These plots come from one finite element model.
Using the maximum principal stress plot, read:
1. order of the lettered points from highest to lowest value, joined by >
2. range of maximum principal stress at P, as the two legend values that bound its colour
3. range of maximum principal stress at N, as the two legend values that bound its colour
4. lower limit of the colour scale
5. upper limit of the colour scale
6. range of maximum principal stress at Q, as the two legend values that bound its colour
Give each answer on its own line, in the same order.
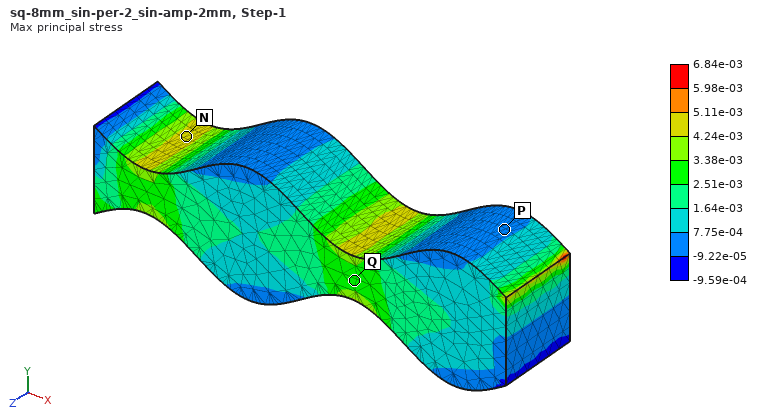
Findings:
N > Q > P
-9.22e-05 to 7.75e-04
4.24e-03 to 5.11e-03
-9.59e-04
6.84e-03
2.51e-03 to 3.38e-03
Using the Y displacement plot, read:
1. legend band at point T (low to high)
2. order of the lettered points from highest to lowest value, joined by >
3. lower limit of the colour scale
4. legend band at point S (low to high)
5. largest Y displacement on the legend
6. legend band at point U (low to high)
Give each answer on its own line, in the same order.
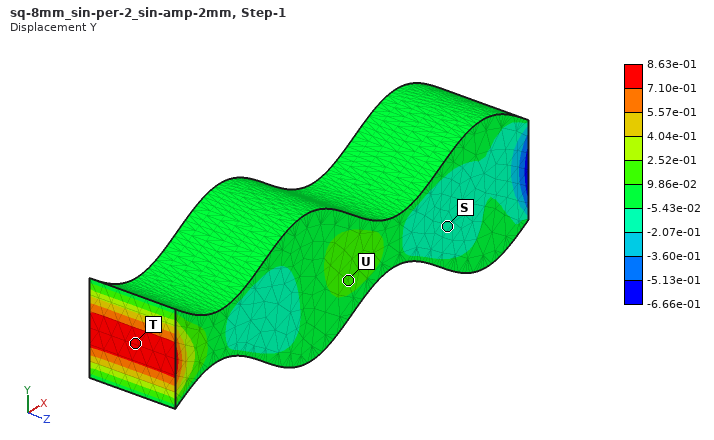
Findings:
7.10e-01 to 8.63e-01
T > U > S
-6.66e-01
-2.07e-01 to -5.43e-02
8.63e-01
9.86e-02 to 2.52e-01
